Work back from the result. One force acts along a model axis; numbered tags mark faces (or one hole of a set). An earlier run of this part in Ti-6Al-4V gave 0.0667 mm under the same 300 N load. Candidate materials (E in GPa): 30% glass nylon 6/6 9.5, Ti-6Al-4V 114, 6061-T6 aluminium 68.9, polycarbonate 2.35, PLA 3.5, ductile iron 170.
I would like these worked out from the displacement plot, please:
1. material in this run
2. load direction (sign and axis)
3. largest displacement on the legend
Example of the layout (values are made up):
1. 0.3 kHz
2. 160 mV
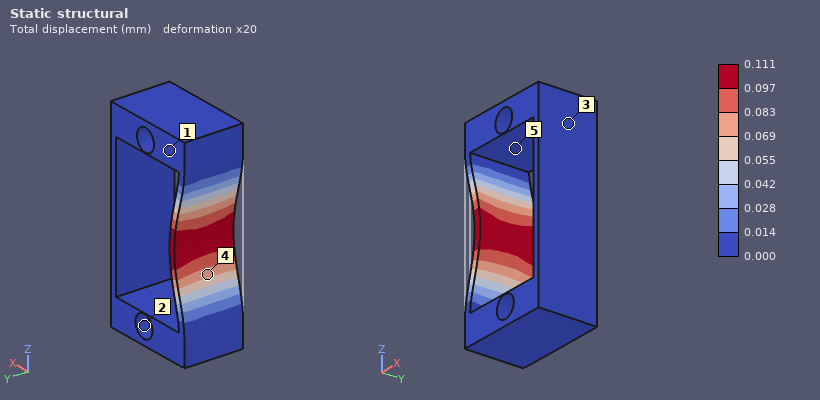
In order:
1. 6061-T6 aluminium
2. +X
3. 0.111 mm
